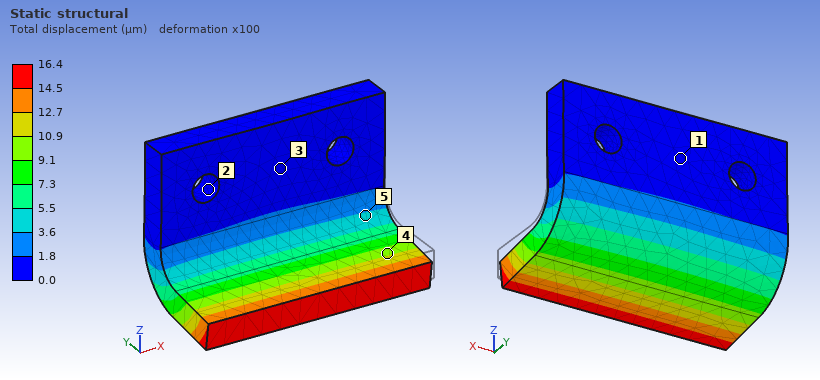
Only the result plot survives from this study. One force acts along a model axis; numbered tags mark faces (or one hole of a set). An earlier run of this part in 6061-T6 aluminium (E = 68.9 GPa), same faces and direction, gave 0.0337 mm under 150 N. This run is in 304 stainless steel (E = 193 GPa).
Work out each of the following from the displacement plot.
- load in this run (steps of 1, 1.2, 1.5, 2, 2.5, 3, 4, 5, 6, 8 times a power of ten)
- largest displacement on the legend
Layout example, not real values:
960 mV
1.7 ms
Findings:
200 N
16.4 µm
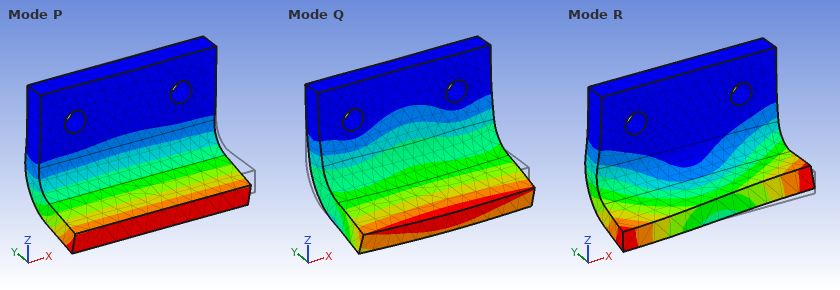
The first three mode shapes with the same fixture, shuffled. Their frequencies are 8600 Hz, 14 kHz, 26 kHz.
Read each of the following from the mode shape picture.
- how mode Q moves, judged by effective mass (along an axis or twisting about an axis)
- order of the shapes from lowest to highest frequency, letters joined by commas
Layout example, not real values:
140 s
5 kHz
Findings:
along Y
P, R, Q
